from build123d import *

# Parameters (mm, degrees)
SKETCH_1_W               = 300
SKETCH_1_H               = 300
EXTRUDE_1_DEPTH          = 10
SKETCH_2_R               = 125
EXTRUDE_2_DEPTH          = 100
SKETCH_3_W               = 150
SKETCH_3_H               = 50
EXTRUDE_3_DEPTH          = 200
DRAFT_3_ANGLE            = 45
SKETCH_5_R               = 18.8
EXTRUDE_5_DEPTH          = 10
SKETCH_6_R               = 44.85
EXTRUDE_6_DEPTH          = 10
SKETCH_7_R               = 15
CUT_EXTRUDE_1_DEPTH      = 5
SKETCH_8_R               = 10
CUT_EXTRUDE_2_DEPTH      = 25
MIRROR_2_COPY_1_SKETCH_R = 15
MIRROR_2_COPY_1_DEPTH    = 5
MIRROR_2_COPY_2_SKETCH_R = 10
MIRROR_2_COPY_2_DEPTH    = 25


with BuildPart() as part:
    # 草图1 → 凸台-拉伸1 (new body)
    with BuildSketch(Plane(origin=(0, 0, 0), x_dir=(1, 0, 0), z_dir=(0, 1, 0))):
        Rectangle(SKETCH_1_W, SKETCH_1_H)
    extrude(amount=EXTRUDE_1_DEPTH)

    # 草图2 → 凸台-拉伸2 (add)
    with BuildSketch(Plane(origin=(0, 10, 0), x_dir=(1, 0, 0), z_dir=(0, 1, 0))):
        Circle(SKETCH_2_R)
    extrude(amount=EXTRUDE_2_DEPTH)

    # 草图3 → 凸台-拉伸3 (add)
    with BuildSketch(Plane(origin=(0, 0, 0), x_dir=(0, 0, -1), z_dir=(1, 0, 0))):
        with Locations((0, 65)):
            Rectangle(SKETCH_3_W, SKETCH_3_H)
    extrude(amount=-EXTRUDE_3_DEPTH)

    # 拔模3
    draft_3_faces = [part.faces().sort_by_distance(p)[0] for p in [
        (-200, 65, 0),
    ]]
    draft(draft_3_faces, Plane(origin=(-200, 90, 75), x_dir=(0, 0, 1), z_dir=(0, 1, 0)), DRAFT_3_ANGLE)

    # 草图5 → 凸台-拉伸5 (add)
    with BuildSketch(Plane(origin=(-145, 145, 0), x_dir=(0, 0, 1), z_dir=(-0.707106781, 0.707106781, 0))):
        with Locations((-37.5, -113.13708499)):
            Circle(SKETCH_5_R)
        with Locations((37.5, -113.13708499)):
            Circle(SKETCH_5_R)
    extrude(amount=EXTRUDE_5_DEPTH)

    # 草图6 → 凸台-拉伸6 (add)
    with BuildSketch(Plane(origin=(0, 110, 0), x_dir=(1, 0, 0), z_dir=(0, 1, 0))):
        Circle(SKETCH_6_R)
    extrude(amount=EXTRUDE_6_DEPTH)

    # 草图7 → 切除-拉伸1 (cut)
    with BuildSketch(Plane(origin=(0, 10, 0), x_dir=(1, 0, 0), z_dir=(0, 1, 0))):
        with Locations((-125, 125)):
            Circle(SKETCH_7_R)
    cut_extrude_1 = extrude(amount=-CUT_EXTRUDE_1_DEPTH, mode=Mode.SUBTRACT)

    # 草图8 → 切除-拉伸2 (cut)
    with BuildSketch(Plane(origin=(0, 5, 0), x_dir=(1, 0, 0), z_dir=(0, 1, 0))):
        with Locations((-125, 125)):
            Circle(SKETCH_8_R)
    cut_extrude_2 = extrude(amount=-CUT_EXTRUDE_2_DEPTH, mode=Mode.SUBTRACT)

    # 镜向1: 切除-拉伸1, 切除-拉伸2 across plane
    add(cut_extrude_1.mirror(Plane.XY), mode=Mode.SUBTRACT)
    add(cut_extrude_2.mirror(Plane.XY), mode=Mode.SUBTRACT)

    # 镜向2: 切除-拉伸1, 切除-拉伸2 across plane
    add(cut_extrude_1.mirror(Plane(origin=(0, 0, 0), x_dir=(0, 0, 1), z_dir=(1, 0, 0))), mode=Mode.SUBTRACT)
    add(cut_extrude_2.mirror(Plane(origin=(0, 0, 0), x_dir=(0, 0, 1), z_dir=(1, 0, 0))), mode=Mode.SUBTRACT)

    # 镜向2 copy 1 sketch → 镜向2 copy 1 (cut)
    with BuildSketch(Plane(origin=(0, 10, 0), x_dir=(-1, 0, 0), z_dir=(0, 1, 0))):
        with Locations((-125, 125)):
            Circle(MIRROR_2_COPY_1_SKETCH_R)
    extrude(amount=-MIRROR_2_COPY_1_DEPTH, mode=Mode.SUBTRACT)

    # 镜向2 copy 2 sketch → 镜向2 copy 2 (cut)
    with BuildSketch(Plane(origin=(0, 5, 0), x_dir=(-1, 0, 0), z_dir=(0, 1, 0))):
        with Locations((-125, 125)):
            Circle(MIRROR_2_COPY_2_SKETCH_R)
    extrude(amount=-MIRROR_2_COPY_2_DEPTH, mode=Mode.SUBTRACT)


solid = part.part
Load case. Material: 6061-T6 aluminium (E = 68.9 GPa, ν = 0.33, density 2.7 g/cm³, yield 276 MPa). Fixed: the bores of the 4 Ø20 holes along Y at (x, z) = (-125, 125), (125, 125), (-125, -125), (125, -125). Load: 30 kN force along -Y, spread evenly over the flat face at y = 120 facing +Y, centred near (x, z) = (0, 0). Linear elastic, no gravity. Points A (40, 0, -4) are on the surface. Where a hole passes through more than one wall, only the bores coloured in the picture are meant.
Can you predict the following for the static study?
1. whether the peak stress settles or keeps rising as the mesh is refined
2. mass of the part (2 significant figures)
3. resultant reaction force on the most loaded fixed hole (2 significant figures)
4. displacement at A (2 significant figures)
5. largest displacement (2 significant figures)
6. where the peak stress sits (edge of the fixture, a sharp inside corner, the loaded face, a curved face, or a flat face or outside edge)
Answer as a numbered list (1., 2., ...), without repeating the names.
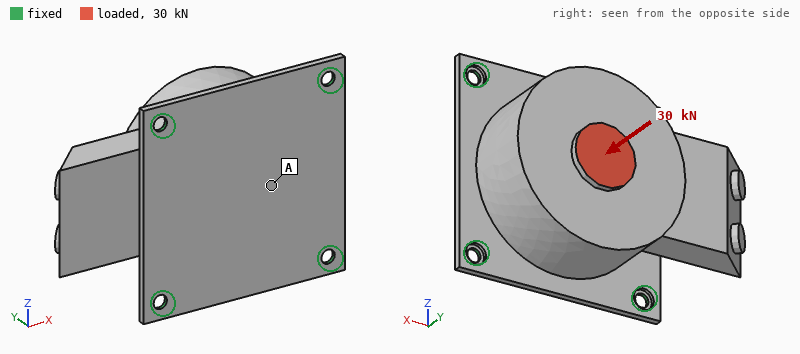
1. keeps rising
2. 18 kg
3. 14 kN
4. 0.29 mm
5. 0.29 mm
6. edge of the fixture
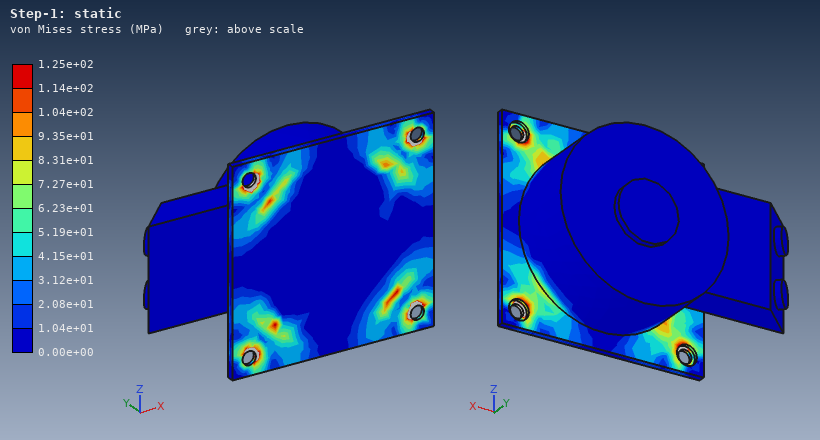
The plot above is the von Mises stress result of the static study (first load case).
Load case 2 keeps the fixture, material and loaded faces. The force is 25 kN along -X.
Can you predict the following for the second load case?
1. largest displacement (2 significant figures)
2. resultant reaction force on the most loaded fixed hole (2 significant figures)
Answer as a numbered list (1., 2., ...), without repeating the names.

1. 0.57 mm
2. 12 kN
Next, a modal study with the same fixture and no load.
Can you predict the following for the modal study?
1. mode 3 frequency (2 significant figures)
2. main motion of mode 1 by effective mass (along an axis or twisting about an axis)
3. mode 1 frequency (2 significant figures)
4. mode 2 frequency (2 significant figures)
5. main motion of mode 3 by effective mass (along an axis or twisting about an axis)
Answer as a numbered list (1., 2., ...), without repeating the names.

1. 500 Hz
2. along Y
3. 360 Hz
4. 450 Hz
5. along Z
